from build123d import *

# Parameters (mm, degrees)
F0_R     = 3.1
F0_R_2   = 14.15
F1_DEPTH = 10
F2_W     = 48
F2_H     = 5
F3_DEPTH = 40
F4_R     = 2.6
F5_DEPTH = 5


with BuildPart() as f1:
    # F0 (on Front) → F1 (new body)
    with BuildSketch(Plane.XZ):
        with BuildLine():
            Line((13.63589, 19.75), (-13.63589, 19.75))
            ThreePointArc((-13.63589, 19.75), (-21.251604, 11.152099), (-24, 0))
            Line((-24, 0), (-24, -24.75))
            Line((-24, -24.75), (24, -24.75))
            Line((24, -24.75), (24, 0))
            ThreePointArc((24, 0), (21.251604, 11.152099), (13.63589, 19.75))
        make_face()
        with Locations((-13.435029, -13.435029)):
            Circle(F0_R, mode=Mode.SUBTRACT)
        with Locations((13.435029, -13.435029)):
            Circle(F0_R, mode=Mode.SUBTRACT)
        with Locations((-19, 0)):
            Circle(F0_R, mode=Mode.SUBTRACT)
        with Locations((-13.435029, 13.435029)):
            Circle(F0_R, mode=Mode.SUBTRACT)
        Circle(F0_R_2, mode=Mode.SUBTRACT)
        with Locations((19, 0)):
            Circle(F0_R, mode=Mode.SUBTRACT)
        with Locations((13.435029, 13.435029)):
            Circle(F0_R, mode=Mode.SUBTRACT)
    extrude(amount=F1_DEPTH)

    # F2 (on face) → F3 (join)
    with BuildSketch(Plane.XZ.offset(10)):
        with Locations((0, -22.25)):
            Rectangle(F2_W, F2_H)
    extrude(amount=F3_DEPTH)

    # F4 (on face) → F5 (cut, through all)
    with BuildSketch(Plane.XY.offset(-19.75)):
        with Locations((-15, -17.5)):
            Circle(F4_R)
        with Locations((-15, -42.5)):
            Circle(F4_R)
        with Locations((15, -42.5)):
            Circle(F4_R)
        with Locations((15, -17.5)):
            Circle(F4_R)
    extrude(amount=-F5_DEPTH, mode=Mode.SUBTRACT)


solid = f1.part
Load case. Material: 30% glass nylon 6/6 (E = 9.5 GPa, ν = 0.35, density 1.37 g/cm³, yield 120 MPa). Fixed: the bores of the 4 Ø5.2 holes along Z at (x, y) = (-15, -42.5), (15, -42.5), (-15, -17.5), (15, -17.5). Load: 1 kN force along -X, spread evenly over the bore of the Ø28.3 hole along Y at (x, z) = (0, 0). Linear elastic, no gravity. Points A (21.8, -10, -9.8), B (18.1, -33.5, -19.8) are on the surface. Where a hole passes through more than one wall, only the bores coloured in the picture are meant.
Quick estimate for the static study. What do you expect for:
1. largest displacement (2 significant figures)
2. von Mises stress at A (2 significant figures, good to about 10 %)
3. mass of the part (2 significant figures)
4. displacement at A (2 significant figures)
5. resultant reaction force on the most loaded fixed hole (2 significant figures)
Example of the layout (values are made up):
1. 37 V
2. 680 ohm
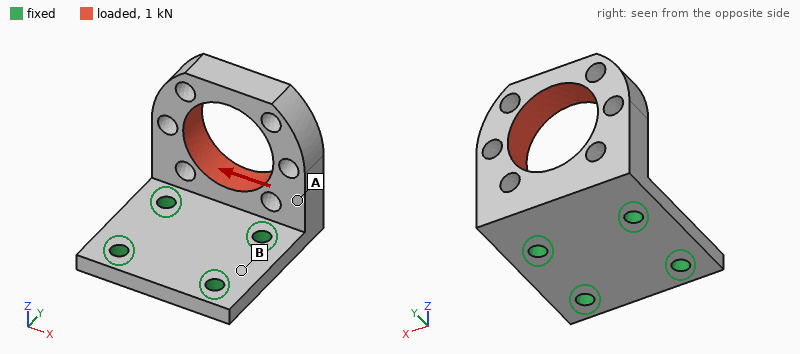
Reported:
1. 0.41 mm
2. 12 MPa
3. 29 g
4. 0.16 mm
5. 890 N
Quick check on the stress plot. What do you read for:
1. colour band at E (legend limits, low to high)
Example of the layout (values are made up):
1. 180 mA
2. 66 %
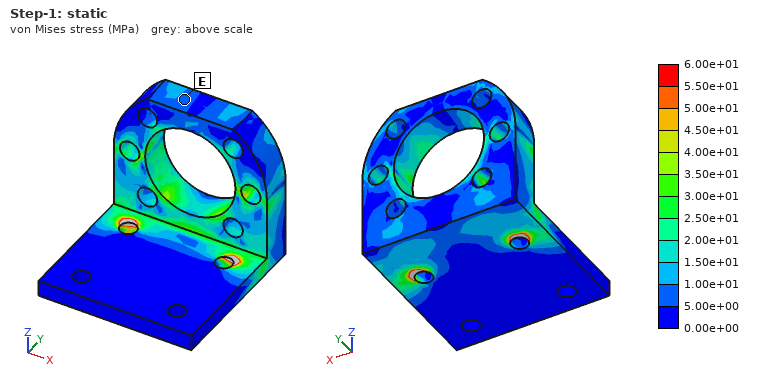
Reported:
1. 5.00e+00 to 1.00e+01 MPa
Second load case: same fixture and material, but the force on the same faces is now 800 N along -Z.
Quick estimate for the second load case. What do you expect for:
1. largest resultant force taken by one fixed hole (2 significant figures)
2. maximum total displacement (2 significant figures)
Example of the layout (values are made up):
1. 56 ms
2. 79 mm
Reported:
1. 440 N
2. 0.53 mm
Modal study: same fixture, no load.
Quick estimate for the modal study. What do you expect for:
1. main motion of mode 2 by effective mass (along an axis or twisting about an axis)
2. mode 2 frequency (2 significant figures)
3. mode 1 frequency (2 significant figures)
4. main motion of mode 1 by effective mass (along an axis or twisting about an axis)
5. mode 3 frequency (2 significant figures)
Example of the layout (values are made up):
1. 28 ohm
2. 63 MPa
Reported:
1. along X
2. 2400 Hz
3. 1100 Hz
4. along Y
5. 3600 Hz
